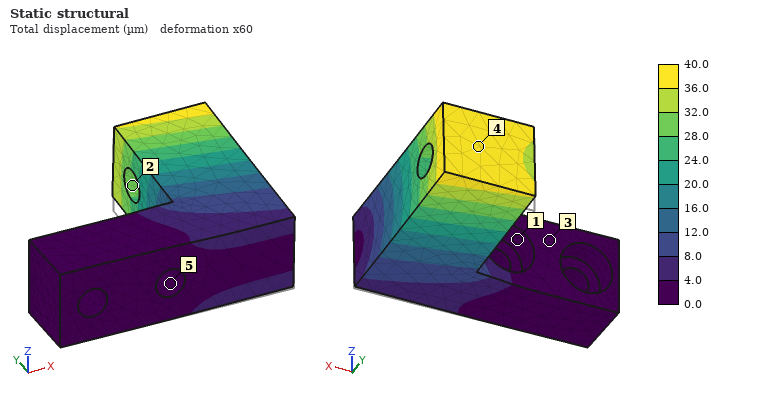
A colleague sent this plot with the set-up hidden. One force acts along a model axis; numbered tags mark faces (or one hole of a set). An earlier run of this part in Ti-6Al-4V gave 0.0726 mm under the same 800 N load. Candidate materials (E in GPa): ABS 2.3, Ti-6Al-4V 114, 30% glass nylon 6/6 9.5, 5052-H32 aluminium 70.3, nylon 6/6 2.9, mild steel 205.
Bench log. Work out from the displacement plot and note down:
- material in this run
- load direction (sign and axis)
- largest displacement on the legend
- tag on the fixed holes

mild steel
+Z
40.0 µm
5
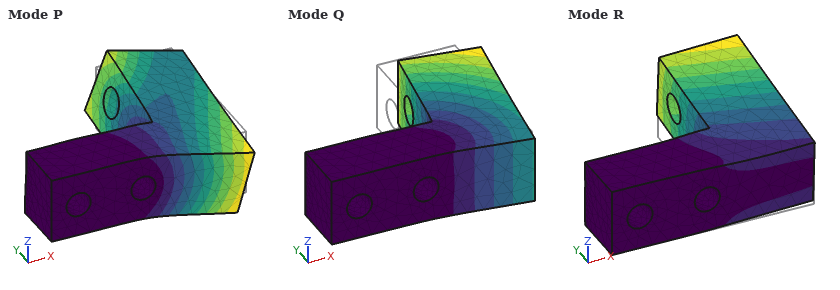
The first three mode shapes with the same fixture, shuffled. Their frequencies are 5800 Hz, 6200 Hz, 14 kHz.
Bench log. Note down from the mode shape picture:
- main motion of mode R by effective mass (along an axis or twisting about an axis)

along Z
